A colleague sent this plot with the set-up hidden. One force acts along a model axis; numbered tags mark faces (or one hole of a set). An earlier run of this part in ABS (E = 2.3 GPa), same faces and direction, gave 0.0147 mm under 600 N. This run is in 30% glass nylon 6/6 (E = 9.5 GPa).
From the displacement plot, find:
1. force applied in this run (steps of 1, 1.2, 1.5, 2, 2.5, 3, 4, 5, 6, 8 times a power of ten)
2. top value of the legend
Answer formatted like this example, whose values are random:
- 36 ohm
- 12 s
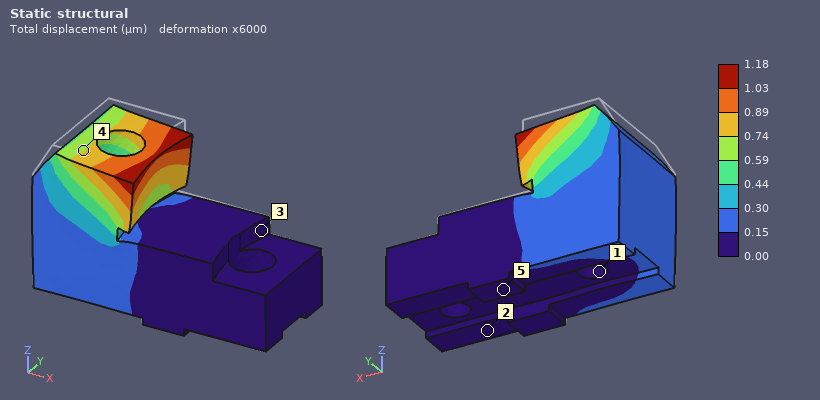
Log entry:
- 200 N
- 1.18 µm
